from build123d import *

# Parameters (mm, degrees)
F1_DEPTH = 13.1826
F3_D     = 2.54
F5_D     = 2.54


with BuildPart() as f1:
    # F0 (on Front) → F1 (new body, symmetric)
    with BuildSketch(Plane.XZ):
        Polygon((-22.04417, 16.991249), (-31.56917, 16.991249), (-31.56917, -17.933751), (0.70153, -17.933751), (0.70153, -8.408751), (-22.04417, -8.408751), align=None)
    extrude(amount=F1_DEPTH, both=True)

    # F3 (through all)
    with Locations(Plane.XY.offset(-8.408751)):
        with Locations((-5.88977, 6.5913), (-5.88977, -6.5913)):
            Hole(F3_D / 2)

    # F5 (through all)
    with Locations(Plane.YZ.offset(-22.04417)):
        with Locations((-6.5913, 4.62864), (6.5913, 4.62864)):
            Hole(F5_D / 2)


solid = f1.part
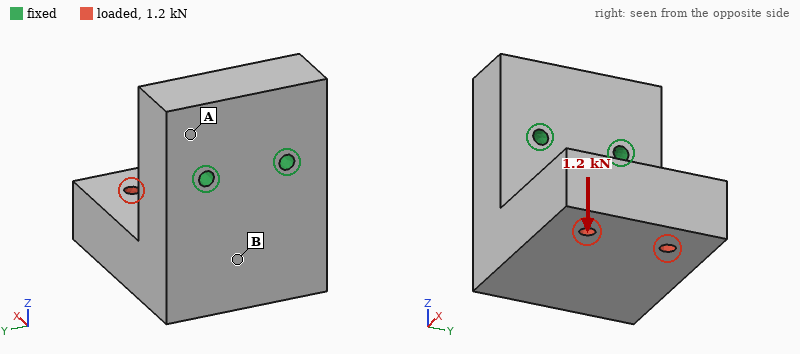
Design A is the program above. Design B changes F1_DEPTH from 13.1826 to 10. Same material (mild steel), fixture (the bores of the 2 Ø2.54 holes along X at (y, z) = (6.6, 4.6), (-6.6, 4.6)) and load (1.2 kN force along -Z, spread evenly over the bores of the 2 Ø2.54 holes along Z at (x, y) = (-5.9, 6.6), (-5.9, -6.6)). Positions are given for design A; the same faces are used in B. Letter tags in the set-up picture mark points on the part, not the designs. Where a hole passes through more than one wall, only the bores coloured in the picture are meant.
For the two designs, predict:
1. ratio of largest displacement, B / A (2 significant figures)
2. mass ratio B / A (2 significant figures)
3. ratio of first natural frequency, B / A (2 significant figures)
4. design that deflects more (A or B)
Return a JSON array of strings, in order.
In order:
["1.3", "0.76", "1.0", "B"]
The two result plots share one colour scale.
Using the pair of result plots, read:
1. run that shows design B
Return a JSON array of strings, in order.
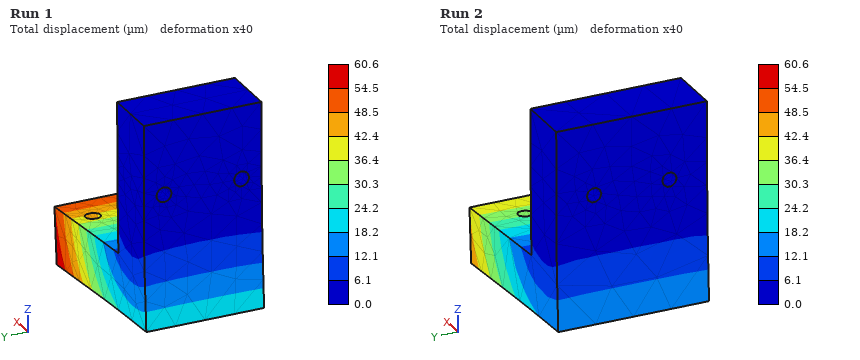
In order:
["Run 1"]
